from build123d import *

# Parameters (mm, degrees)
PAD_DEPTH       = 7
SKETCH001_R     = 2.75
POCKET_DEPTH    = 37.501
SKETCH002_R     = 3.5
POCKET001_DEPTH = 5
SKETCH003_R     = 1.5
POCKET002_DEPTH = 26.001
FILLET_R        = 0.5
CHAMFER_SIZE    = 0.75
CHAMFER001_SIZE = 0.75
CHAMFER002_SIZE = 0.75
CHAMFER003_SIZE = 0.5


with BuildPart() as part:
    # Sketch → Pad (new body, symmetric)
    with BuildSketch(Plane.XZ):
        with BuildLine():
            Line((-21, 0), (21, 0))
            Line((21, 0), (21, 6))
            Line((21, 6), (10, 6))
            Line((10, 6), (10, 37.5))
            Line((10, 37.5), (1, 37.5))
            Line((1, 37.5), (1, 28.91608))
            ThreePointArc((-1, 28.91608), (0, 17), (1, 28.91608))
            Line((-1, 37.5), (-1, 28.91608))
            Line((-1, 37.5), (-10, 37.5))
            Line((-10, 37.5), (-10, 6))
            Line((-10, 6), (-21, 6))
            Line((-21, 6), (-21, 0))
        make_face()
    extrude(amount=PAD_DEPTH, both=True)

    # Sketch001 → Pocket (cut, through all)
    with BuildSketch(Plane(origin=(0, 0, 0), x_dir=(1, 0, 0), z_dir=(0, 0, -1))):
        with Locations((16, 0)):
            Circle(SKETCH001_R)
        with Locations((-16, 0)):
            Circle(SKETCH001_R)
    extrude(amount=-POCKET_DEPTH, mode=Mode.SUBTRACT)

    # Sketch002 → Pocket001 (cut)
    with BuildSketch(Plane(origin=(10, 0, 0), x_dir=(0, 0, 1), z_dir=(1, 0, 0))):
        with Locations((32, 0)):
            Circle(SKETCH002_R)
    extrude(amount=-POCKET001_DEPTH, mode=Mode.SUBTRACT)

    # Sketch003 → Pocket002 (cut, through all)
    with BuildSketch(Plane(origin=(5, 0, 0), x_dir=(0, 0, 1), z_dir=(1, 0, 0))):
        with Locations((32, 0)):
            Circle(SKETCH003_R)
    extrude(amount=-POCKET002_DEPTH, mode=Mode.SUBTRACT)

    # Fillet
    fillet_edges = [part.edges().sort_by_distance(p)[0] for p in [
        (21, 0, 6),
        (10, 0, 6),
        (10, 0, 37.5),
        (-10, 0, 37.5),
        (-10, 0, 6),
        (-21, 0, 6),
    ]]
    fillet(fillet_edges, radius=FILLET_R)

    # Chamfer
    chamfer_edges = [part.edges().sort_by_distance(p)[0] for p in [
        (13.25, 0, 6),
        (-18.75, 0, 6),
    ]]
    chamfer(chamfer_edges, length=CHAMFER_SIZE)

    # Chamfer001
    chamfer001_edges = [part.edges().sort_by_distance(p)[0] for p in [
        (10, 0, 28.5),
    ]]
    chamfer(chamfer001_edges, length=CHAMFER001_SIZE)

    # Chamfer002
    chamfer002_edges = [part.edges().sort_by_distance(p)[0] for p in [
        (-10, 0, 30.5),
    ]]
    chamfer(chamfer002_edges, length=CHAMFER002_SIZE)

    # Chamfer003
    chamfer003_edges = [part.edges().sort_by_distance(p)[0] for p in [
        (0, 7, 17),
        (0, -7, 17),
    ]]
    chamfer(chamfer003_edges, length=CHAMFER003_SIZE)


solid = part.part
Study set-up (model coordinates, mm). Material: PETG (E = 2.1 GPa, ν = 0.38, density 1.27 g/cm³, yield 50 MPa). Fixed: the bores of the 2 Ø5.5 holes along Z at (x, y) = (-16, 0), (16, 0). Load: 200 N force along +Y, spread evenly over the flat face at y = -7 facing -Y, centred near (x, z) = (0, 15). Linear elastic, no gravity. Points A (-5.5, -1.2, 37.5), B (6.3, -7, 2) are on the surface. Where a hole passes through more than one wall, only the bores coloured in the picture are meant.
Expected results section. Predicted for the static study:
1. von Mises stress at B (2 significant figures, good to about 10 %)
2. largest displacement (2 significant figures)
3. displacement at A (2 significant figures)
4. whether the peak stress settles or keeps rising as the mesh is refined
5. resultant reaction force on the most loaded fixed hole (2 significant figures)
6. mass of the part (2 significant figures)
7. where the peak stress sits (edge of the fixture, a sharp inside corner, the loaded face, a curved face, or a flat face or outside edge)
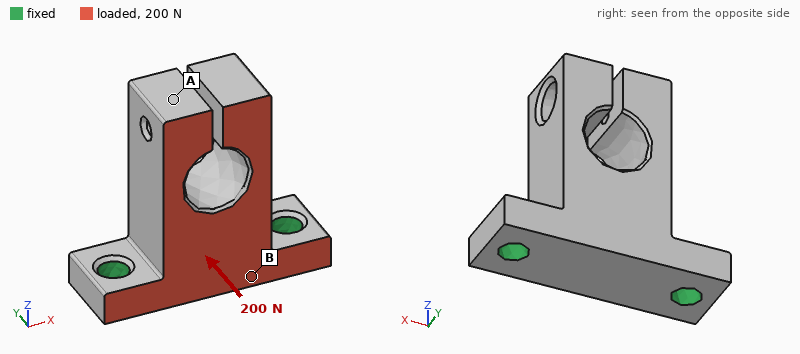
2.7 MPa
0.53 mm
0.51 mm
keeps rising
100 N
13 g
edge of the fixture
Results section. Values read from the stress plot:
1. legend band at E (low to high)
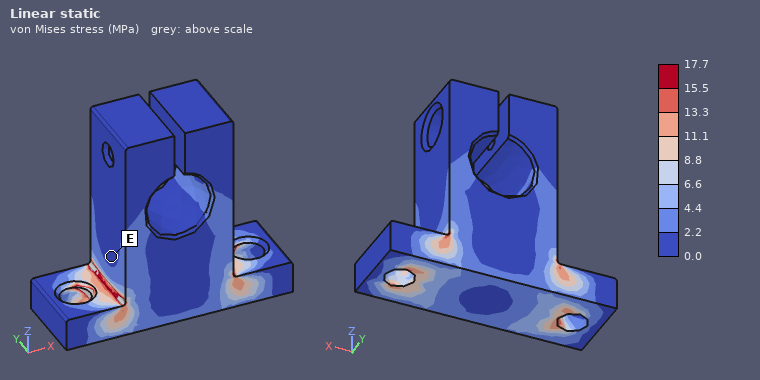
0.0 to 2.2 MPa
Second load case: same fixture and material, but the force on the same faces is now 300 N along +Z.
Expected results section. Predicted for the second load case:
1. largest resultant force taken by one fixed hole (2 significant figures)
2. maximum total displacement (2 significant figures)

160 N
0.41 mm
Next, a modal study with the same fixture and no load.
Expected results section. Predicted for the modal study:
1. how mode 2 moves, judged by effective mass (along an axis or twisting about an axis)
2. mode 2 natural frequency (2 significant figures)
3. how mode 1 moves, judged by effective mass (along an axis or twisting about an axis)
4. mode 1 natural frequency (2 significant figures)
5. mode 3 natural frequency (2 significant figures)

along X
1400 Hz
along Y
1100 Hz
1500 Hz
